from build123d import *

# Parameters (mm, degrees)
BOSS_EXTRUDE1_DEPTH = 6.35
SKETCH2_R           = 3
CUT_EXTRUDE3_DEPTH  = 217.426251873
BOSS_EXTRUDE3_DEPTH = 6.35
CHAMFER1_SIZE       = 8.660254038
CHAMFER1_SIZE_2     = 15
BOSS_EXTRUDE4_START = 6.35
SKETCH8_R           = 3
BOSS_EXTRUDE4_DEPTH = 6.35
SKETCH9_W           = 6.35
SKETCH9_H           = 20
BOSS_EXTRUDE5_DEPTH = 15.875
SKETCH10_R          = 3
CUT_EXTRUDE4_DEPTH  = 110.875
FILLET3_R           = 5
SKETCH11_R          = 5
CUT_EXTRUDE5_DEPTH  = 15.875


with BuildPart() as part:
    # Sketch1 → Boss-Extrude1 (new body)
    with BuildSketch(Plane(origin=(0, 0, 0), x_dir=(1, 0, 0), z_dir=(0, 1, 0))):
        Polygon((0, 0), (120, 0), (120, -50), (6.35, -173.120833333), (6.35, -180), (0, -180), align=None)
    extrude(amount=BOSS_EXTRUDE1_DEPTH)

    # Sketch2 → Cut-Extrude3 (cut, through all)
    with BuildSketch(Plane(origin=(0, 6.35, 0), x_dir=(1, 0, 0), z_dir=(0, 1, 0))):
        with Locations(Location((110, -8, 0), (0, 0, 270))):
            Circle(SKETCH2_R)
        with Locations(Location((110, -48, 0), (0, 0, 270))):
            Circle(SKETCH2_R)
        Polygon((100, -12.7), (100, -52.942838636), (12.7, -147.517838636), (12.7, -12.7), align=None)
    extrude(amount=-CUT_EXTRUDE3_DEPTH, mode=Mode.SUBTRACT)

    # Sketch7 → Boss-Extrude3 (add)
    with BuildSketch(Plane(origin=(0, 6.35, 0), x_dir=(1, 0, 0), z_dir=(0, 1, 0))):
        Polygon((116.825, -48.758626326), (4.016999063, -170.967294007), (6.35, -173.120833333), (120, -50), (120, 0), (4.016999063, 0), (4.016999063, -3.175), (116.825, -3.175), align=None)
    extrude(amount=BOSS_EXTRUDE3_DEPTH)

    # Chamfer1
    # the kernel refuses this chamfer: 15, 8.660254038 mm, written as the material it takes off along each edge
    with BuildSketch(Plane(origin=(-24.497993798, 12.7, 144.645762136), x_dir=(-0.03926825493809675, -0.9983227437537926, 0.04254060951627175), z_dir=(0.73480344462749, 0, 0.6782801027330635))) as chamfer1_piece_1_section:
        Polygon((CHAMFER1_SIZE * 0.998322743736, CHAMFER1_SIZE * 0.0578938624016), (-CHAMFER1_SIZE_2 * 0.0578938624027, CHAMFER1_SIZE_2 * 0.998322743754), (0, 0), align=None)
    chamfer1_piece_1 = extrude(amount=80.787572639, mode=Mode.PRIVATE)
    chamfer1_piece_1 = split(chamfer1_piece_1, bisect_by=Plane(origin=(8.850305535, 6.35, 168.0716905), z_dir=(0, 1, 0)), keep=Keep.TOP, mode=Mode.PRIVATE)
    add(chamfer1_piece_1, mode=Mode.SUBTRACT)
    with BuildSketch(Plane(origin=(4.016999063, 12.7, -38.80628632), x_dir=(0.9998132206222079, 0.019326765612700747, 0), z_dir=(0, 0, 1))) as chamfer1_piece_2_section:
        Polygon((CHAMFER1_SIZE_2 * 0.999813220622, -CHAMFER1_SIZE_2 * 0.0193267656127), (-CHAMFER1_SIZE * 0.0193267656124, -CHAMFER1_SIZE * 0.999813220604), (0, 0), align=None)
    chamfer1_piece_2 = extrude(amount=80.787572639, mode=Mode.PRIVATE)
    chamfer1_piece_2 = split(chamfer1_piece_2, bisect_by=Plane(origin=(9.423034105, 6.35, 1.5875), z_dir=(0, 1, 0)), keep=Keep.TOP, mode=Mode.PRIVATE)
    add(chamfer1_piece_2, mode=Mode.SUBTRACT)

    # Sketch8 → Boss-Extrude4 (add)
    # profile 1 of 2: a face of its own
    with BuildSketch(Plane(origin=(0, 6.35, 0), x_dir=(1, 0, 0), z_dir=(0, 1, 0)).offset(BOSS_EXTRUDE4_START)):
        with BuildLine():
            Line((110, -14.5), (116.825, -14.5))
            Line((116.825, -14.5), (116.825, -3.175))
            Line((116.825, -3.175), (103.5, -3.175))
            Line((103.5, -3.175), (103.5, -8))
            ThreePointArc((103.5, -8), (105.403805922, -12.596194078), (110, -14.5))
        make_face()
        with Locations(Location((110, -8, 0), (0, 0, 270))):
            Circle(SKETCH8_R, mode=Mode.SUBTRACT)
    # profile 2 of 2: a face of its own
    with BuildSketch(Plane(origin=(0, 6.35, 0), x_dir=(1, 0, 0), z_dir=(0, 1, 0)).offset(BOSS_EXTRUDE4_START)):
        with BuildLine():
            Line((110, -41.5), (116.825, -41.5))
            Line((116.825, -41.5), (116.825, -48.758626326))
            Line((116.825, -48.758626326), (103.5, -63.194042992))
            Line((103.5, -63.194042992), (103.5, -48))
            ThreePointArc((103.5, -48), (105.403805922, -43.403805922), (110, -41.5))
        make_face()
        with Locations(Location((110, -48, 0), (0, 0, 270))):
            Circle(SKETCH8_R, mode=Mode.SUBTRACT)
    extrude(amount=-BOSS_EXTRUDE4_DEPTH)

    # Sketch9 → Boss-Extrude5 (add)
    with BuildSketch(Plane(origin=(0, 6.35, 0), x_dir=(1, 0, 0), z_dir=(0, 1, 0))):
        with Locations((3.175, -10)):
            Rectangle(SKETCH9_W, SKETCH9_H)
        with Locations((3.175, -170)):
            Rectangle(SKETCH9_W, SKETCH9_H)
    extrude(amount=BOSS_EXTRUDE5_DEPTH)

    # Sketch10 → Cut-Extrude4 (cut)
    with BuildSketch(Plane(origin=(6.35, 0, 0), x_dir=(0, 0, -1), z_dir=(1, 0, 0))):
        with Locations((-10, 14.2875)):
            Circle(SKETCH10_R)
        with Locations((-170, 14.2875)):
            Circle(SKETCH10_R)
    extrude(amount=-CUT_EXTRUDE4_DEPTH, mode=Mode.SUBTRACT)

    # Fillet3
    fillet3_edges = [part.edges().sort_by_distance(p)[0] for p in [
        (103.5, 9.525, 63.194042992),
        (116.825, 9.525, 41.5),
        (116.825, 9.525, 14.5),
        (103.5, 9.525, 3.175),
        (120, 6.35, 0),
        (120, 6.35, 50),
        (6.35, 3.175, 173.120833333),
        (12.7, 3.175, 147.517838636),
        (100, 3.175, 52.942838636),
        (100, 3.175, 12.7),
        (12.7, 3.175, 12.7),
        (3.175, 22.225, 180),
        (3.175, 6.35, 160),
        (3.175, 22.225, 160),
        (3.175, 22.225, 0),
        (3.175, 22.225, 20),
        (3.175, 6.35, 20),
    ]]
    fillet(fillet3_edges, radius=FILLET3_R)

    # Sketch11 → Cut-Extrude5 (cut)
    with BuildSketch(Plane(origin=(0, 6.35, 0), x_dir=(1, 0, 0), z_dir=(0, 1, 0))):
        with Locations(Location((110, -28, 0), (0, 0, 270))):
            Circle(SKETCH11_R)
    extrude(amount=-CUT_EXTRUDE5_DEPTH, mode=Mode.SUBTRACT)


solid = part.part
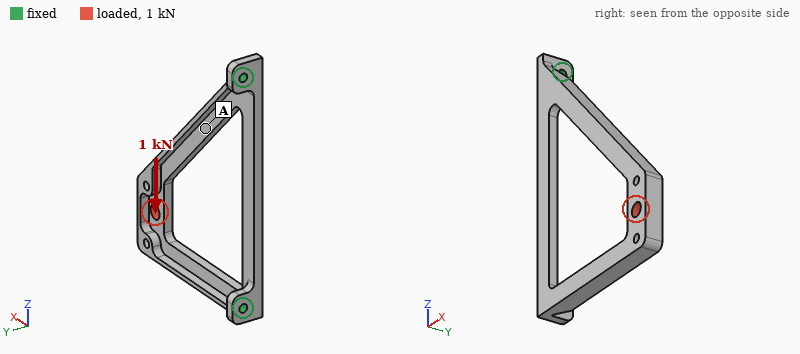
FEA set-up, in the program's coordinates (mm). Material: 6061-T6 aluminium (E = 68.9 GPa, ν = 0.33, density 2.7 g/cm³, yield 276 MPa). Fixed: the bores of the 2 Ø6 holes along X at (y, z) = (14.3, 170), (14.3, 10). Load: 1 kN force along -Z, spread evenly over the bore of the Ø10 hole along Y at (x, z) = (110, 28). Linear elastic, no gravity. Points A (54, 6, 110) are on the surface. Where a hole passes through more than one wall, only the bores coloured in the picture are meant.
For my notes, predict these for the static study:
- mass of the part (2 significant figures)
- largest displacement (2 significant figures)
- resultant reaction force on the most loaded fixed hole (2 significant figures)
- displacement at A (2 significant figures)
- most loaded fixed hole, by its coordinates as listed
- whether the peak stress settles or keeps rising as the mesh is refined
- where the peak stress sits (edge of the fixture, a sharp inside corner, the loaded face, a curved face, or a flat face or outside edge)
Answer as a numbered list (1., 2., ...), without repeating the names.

1. 140 g
2. 0.27 mm
3. 930 N
4. 0.15 mm
5. (14.3, 170)
6. keeps rising
7. edge of the fixture
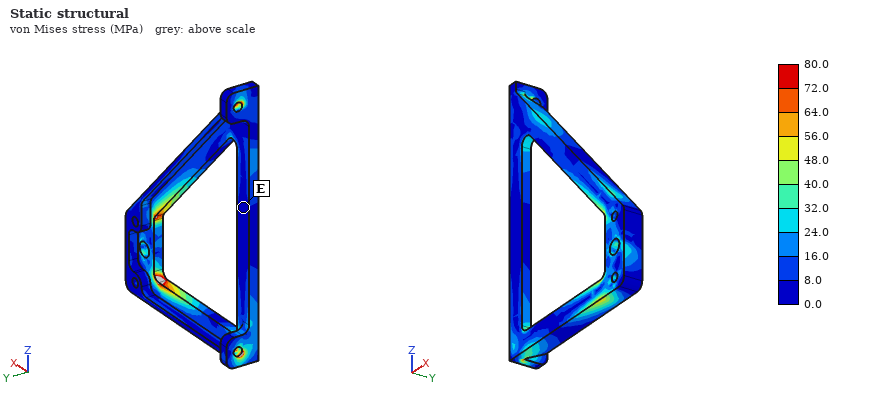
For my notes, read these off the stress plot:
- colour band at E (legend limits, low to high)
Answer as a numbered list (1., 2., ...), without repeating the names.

1. 0.0 to 8.0 MPa
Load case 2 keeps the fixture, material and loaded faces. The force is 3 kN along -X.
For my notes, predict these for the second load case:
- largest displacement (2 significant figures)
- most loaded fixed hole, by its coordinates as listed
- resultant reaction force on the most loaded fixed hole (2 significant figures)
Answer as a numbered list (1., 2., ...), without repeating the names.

1. 0.67 mm
2. (14.3, 10)
3. 2.5 kN
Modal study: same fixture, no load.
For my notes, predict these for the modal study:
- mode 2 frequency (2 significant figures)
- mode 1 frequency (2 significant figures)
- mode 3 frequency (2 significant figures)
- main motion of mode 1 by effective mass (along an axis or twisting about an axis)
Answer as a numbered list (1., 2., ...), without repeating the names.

1. 920 Hz
2. 270 Hz
3. 1300 Hz
4. along Y
